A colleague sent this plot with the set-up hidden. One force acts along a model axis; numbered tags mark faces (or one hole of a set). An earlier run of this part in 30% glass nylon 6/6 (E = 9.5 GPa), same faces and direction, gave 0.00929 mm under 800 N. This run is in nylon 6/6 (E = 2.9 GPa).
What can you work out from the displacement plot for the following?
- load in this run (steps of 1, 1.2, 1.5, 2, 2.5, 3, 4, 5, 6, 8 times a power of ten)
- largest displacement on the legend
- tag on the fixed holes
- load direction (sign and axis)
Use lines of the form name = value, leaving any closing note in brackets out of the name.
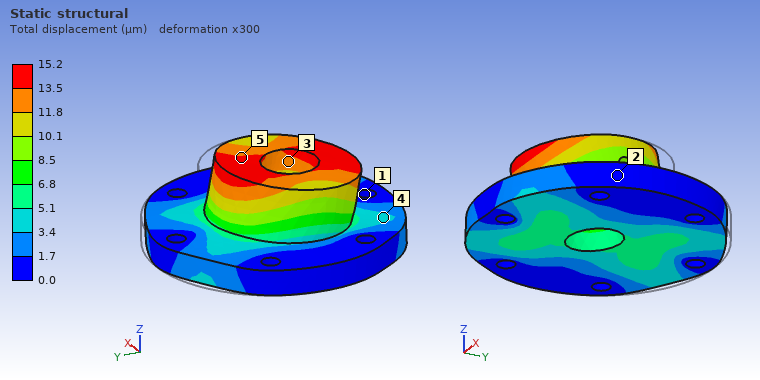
load in this run = 400 N
largest displacement on the legend = 15.2 µm
tag on the fixed holes = 1
load direction = -Y
